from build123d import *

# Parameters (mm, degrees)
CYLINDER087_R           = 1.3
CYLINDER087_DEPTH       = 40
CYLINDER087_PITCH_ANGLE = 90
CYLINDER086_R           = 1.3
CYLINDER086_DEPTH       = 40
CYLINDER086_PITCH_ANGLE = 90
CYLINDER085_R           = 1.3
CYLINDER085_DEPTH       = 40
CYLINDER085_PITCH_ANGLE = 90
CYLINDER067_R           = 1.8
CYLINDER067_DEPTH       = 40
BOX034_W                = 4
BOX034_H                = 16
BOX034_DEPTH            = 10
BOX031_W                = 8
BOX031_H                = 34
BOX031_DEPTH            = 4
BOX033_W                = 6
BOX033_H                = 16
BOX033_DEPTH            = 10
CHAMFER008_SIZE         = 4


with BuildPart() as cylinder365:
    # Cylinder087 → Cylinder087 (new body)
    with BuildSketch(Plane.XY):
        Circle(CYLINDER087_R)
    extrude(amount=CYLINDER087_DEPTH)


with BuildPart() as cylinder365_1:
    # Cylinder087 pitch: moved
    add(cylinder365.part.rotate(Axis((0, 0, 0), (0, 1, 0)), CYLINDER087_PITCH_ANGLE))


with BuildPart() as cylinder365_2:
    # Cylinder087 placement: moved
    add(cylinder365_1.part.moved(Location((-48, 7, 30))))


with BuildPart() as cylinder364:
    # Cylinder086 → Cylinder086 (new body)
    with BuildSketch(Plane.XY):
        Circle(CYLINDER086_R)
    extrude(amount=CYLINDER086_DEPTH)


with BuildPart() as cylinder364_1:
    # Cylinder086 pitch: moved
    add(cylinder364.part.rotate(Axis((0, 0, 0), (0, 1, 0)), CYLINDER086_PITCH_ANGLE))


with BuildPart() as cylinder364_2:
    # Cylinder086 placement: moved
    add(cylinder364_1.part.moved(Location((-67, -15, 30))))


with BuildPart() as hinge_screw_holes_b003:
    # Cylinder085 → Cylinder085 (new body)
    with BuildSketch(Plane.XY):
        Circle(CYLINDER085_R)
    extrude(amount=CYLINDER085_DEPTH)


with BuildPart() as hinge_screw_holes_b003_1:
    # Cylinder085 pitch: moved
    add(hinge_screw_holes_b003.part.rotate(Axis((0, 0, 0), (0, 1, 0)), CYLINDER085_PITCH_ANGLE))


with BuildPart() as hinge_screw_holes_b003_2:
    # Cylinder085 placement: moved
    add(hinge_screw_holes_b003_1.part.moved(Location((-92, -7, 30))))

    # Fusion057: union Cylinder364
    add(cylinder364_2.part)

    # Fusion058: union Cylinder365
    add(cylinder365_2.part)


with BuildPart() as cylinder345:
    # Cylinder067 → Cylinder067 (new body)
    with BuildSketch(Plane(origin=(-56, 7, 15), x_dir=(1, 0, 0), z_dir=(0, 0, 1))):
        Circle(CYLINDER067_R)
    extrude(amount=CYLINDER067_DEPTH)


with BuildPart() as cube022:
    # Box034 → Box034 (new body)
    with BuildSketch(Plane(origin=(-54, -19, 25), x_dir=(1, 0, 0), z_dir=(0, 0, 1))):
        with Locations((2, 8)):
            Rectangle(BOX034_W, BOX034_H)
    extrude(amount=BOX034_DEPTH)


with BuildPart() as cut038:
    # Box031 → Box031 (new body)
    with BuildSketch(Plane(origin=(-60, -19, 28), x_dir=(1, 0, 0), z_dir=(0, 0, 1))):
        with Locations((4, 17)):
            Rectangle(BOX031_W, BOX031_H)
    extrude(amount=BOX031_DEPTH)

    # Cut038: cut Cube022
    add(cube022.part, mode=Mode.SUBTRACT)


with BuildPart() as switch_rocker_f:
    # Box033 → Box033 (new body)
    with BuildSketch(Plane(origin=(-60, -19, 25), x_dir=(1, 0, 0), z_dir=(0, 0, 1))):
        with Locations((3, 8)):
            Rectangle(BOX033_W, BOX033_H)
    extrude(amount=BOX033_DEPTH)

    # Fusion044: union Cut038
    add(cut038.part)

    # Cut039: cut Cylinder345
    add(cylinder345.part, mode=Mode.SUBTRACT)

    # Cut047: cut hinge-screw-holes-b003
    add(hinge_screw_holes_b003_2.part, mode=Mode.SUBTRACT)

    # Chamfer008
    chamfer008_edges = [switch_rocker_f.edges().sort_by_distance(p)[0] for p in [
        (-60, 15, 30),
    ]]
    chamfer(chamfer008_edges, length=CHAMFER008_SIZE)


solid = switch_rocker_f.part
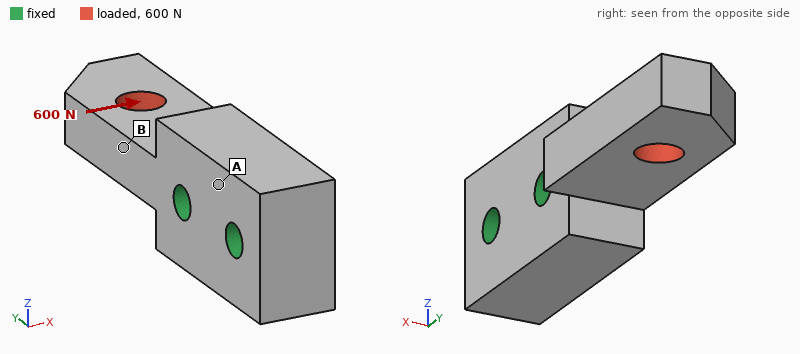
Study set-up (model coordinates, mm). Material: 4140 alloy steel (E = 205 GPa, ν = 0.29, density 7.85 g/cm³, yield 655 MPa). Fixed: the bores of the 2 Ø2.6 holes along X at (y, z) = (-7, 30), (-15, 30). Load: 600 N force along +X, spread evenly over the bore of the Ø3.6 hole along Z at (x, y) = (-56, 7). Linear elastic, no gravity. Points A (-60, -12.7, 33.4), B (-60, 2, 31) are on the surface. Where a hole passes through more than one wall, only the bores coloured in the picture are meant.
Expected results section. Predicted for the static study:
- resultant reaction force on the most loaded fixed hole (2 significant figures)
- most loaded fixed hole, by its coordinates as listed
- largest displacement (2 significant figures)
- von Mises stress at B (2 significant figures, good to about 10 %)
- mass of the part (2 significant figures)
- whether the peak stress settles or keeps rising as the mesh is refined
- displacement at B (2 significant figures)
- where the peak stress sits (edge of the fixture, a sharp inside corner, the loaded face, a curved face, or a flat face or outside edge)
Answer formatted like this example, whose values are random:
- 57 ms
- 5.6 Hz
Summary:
- 760 N
- (-7, 30)
- 49 µm
- 83 MPa
- 11 g
- keeps rising
- 15 µm
- edge of the fixture
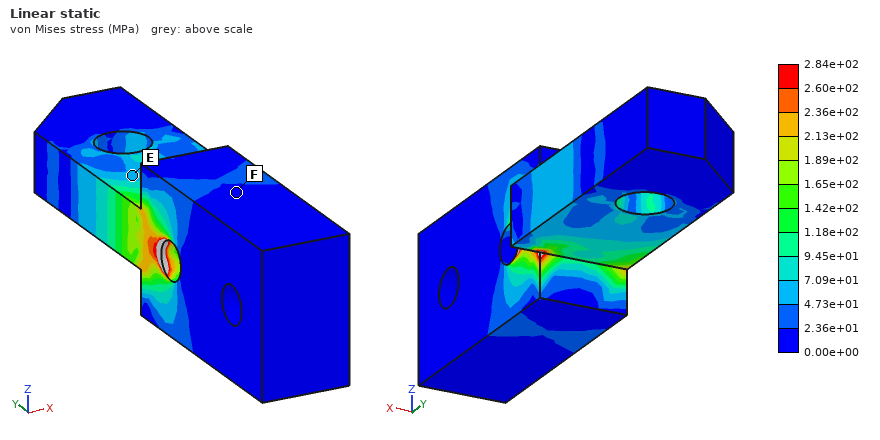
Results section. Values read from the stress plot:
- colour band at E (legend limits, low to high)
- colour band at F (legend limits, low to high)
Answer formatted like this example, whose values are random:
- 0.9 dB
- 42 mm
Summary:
- 4.73e+01 to 7.09e+01 MPa
- 0.00e+00 to 2.36e+01 MPa
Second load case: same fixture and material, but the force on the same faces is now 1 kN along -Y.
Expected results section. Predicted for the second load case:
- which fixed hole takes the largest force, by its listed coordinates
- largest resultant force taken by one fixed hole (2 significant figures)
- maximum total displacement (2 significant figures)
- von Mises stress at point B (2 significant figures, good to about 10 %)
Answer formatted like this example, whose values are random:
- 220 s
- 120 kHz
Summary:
- (-7, 30)
- 900 N
- 6.5 µm
- 32 MPa
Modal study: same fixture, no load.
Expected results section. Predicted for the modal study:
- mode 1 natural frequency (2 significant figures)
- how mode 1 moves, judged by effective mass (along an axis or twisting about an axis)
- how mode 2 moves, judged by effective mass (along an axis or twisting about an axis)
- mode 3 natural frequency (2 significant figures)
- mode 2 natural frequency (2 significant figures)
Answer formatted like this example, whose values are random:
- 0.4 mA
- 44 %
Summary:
- 8500 Hz
- along Z
- along X
- 31 kHz
- 12 kHz
